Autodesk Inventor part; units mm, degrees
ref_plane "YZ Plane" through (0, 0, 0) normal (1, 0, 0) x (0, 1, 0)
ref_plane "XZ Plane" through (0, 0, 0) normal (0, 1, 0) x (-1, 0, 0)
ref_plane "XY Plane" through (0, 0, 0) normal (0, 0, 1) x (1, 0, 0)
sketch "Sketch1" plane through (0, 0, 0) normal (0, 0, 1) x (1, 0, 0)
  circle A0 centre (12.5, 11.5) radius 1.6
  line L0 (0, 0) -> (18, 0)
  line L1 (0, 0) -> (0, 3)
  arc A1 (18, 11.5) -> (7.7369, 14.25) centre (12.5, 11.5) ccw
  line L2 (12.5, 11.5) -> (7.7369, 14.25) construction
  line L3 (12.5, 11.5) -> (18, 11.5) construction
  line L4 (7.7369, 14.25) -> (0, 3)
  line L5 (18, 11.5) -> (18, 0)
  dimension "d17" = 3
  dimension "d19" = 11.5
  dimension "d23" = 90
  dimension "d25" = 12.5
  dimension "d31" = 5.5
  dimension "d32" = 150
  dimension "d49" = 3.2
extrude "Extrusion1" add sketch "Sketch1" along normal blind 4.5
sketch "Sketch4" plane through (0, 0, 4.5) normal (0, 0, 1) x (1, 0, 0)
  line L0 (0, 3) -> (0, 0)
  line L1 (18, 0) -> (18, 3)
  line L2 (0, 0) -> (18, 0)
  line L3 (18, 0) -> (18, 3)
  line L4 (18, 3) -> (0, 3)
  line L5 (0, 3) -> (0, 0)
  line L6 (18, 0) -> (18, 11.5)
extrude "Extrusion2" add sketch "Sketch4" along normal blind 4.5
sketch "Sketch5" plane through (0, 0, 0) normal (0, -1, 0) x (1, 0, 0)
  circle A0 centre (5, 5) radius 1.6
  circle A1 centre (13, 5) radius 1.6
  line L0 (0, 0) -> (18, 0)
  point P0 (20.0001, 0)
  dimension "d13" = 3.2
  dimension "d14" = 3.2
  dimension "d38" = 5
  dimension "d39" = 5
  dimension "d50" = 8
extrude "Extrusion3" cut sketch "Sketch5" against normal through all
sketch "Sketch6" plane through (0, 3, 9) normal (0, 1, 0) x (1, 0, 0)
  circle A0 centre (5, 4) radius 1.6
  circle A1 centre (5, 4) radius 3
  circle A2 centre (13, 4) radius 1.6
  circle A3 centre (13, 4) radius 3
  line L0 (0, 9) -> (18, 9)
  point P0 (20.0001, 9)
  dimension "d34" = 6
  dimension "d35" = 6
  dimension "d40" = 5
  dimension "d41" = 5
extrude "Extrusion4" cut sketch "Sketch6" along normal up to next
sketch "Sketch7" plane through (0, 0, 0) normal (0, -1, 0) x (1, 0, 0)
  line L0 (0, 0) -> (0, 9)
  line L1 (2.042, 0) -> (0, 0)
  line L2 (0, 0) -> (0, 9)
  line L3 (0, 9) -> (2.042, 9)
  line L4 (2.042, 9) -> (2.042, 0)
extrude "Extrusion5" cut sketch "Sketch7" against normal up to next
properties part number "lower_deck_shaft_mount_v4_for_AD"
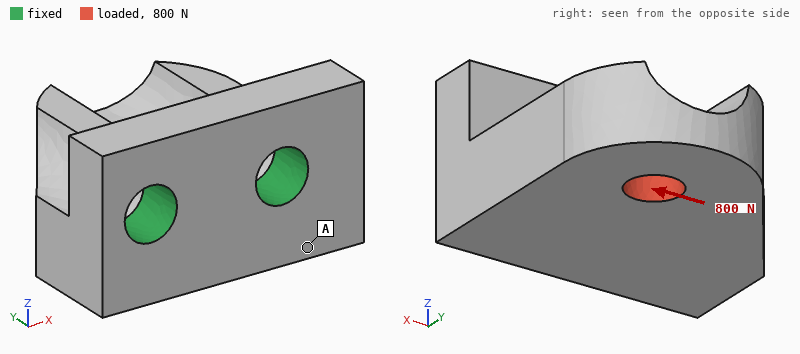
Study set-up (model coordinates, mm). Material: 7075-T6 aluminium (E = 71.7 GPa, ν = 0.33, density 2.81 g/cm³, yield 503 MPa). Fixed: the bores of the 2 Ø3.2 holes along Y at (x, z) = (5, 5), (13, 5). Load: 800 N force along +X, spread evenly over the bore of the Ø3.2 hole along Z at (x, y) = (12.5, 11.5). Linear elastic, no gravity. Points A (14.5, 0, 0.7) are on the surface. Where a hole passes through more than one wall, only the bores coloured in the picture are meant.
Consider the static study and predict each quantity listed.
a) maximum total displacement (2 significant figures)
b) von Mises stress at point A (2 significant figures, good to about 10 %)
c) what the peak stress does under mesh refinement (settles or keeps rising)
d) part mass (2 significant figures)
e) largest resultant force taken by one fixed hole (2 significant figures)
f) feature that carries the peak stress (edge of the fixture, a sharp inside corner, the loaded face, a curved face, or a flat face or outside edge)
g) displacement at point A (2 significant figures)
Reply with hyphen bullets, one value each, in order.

- 44 µm
- 26 MPa
- keeps rising
- 2.6 g
- 880 N
- edge of the fixture
- 8.0 µm
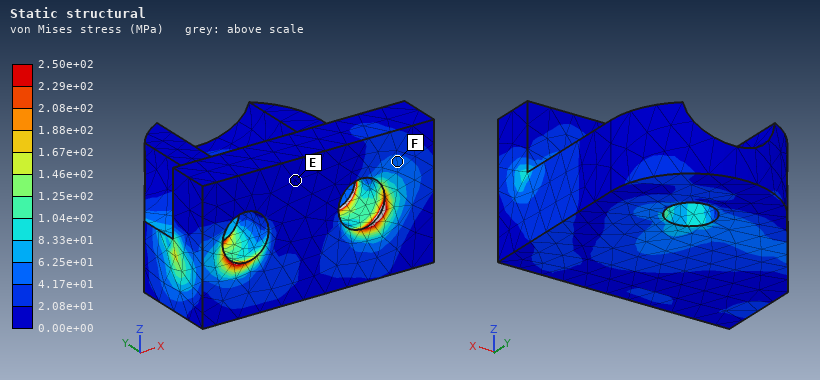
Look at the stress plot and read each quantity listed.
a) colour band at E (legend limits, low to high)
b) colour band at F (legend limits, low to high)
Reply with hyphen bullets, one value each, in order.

- 0.00e+00 to 2.08e+01 MPa
- 4.17e+01 to 6.25e+01 MPa
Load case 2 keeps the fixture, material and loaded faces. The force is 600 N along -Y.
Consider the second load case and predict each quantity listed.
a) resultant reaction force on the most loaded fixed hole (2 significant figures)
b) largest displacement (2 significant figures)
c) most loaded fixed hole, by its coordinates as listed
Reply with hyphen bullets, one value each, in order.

- 490 N
- 31 µm
- (13, 5)
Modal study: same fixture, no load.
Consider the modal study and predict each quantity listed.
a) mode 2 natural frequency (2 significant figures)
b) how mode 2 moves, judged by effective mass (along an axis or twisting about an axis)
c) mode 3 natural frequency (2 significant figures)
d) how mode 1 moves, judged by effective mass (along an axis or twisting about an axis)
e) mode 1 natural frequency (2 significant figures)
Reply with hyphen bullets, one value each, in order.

- 24 kHz
- along X
- 34 kHz
- along Z
- 13 kHz
